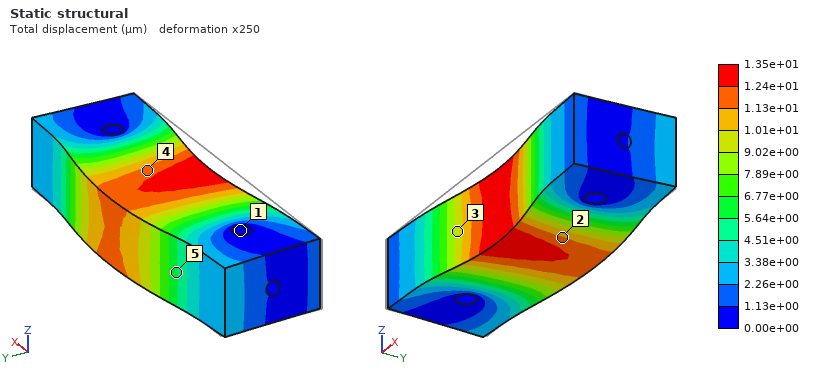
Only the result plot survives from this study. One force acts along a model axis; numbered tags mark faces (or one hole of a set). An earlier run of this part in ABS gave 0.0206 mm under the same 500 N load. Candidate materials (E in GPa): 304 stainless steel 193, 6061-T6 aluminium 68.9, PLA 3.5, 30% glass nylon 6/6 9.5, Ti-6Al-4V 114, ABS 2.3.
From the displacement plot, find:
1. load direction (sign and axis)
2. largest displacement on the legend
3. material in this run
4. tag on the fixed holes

+Y
1.35e+01 µm
PLA
1
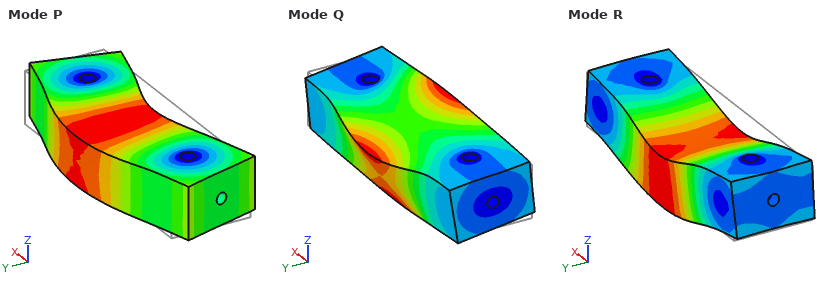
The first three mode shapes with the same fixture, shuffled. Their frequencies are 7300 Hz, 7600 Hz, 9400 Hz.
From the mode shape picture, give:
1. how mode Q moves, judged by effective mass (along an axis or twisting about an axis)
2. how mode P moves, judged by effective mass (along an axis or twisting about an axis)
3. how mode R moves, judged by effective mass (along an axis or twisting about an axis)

twisting about X
along Y
along Z
